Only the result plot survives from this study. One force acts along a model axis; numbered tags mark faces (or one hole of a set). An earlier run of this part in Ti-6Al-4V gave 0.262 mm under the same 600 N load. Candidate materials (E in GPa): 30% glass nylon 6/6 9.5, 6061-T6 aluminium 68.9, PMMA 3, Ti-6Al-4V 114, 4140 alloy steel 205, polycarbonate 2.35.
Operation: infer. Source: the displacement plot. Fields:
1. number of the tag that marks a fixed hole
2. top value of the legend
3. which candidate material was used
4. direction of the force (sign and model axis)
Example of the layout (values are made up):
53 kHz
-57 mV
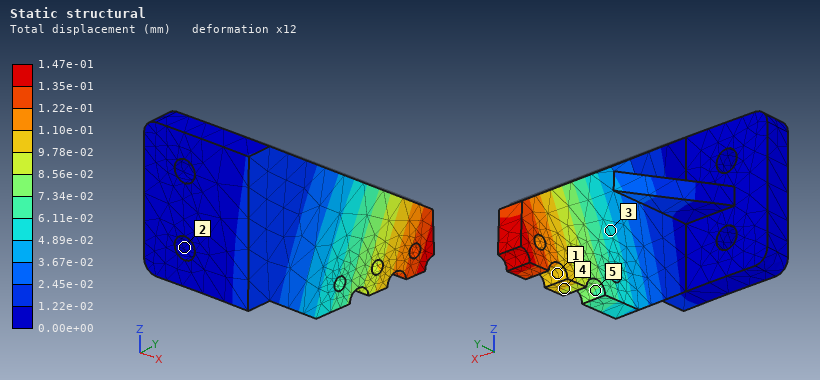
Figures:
2
1.47e-01 mm
4140 alloy steel
+X
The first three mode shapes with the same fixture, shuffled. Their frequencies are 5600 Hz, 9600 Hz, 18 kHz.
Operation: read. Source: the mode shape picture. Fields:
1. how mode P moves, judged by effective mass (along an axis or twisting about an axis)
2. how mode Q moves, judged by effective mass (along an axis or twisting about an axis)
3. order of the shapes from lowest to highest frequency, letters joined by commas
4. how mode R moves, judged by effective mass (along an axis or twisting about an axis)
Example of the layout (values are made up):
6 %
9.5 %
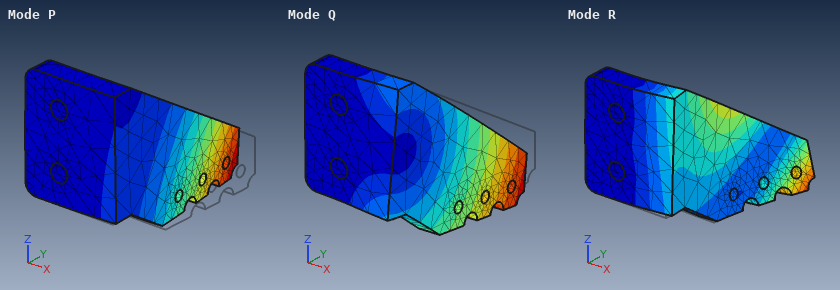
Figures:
along X
along Z
P, Q, R
along Y
